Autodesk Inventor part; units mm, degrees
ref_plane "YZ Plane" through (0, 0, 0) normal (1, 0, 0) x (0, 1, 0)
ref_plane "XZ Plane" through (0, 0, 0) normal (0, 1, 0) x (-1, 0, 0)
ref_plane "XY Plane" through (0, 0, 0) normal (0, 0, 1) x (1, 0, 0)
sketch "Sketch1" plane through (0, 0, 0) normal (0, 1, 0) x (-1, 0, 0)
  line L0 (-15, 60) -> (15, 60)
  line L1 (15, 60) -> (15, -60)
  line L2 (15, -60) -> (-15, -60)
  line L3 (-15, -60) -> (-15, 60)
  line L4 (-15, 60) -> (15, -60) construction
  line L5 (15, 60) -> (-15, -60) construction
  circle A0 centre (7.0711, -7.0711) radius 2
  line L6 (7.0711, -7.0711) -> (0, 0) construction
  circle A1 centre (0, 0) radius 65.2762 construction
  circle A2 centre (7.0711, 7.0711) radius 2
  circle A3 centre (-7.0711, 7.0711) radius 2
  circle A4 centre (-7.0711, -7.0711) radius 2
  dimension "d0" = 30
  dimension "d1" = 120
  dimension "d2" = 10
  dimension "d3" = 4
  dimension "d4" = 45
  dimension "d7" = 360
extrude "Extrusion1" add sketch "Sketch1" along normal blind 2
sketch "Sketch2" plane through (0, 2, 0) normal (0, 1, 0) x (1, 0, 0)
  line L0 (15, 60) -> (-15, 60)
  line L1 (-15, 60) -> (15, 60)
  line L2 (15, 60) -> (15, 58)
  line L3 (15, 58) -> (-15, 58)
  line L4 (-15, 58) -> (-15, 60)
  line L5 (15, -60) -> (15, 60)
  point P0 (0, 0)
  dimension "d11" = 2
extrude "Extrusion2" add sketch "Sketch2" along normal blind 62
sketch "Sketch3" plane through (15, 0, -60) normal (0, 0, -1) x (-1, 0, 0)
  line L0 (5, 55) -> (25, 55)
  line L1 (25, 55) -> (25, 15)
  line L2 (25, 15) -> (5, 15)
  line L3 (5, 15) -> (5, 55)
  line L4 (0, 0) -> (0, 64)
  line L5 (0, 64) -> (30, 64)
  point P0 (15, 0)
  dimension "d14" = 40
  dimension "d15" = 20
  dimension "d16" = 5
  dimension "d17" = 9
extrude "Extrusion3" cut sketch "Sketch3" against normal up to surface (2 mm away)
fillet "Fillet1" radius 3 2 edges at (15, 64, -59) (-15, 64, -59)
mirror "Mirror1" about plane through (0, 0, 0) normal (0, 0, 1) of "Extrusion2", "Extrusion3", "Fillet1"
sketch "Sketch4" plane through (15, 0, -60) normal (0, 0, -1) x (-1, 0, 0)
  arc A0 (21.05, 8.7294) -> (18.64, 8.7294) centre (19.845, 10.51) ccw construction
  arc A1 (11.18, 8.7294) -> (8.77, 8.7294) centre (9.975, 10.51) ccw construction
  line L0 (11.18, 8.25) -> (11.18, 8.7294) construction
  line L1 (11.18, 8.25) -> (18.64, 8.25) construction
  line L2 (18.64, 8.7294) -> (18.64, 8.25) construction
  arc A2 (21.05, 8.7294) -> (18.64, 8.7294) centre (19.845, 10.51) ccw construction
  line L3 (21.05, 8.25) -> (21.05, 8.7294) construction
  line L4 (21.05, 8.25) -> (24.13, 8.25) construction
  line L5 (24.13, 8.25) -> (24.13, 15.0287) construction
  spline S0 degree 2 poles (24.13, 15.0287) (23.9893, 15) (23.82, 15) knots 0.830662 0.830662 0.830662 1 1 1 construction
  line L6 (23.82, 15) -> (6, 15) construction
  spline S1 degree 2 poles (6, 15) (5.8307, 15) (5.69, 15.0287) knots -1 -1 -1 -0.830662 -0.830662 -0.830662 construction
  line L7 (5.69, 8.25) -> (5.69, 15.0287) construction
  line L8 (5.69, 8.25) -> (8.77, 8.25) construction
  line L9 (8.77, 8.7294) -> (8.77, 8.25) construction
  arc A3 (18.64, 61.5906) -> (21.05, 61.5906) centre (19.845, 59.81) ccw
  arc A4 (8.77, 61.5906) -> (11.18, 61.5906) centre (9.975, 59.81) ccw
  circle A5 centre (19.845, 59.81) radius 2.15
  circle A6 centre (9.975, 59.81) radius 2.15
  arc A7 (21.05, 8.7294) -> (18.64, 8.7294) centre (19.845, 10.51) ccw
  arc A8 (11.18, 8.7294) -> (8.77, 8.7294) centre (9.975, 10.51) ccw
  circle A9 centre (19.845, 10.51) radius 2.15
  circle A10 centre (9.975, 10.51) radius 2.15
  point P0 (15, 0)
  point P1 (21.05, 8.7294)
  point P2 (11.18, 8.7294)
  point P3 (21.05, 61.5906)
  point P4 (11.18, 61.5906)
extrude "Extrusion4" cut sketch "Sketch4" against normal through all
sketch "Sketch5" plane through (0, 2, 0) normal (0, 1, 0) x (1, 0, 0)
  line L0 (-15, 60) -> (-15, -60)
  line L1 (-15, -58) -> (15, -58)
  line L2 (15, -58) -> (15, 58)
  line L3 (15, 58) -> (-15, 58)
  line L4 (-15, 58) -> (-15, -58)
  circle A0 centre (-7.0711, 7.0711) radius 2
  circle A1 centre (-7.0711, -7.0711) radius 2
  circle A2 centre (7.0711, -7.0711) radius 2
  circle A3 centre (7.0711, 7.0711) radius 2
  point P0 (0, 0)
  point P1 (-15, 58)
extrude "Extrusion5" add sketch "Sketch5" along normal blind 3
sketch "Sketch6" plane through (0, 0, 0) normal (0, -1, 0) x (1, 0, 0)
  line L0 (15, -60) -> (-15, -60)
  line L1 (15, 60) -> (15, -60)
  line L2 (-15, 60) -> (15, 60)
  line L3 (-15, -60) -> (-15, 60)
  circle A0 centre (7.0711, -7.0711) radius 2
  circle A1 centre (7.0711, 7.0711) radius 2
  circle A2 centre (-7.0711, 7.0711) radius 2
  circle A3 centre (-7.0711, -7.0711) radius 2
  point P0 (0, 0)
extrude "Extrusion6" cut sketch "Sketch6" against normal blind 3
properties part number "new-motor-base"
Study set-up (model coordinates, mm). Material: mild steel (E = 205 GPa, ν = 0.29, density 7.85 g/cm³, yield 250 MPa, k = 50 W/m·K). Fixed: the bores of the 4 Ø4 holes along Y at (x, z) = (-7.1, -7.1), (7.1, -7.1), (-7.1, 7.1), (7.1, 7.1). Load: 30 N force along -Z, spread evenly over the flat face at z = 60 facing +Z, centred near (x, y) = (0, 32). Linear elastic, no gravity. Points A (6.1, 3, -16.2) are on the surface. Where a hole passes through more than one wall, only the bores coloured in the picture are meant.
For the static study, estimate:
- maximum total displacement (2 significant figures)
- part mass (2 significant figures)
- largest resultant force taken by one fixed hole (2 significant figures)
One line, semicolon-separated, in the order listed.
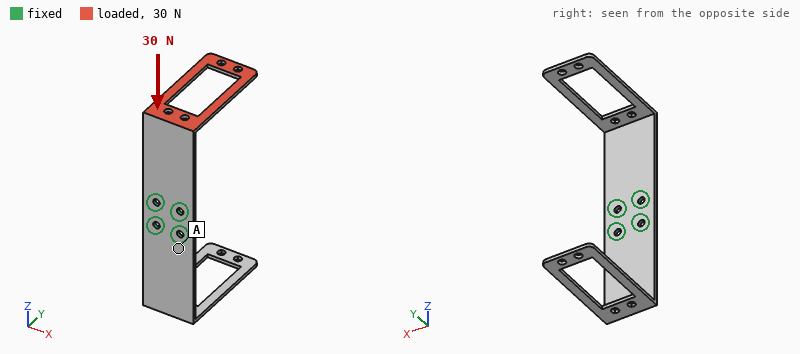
1.1 mm; 84 g; 13 N
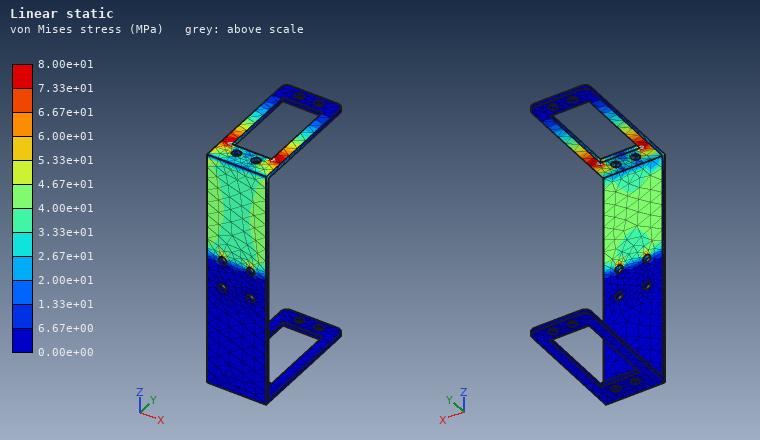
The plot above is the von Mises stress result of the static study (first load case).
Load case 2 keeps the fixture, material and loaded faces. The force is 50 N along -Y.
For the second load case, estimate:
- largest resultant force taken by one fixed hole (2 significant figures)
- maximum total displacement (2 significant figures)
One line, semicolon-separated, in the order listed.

35 N; 1.1 mm
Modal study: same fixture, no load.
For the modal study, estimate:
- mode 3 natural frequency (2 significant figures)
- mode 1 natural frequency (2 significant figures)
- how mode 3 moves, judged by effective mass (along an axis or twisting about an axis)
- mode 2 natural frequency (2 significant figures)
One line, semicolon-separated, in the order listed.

420 Hz; 230 Hz; along X; 230 Hz
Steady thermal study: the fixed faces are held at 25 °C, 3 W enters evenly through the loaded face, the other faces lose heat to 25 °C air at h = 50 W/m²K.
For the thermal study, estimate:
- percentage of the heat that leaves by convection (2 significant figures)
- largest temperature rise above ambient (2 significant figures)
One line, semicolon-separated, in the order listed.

85 %; 29 K
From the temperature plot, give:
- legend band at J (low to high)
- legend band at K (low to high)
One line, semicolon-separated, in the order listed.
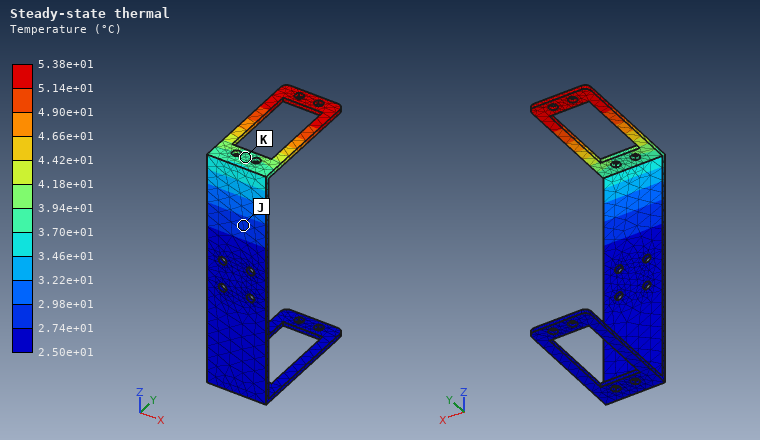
2.74e+01 to 2.98e+01 °C; 3.70e+01 to 3.94e+01 °C
